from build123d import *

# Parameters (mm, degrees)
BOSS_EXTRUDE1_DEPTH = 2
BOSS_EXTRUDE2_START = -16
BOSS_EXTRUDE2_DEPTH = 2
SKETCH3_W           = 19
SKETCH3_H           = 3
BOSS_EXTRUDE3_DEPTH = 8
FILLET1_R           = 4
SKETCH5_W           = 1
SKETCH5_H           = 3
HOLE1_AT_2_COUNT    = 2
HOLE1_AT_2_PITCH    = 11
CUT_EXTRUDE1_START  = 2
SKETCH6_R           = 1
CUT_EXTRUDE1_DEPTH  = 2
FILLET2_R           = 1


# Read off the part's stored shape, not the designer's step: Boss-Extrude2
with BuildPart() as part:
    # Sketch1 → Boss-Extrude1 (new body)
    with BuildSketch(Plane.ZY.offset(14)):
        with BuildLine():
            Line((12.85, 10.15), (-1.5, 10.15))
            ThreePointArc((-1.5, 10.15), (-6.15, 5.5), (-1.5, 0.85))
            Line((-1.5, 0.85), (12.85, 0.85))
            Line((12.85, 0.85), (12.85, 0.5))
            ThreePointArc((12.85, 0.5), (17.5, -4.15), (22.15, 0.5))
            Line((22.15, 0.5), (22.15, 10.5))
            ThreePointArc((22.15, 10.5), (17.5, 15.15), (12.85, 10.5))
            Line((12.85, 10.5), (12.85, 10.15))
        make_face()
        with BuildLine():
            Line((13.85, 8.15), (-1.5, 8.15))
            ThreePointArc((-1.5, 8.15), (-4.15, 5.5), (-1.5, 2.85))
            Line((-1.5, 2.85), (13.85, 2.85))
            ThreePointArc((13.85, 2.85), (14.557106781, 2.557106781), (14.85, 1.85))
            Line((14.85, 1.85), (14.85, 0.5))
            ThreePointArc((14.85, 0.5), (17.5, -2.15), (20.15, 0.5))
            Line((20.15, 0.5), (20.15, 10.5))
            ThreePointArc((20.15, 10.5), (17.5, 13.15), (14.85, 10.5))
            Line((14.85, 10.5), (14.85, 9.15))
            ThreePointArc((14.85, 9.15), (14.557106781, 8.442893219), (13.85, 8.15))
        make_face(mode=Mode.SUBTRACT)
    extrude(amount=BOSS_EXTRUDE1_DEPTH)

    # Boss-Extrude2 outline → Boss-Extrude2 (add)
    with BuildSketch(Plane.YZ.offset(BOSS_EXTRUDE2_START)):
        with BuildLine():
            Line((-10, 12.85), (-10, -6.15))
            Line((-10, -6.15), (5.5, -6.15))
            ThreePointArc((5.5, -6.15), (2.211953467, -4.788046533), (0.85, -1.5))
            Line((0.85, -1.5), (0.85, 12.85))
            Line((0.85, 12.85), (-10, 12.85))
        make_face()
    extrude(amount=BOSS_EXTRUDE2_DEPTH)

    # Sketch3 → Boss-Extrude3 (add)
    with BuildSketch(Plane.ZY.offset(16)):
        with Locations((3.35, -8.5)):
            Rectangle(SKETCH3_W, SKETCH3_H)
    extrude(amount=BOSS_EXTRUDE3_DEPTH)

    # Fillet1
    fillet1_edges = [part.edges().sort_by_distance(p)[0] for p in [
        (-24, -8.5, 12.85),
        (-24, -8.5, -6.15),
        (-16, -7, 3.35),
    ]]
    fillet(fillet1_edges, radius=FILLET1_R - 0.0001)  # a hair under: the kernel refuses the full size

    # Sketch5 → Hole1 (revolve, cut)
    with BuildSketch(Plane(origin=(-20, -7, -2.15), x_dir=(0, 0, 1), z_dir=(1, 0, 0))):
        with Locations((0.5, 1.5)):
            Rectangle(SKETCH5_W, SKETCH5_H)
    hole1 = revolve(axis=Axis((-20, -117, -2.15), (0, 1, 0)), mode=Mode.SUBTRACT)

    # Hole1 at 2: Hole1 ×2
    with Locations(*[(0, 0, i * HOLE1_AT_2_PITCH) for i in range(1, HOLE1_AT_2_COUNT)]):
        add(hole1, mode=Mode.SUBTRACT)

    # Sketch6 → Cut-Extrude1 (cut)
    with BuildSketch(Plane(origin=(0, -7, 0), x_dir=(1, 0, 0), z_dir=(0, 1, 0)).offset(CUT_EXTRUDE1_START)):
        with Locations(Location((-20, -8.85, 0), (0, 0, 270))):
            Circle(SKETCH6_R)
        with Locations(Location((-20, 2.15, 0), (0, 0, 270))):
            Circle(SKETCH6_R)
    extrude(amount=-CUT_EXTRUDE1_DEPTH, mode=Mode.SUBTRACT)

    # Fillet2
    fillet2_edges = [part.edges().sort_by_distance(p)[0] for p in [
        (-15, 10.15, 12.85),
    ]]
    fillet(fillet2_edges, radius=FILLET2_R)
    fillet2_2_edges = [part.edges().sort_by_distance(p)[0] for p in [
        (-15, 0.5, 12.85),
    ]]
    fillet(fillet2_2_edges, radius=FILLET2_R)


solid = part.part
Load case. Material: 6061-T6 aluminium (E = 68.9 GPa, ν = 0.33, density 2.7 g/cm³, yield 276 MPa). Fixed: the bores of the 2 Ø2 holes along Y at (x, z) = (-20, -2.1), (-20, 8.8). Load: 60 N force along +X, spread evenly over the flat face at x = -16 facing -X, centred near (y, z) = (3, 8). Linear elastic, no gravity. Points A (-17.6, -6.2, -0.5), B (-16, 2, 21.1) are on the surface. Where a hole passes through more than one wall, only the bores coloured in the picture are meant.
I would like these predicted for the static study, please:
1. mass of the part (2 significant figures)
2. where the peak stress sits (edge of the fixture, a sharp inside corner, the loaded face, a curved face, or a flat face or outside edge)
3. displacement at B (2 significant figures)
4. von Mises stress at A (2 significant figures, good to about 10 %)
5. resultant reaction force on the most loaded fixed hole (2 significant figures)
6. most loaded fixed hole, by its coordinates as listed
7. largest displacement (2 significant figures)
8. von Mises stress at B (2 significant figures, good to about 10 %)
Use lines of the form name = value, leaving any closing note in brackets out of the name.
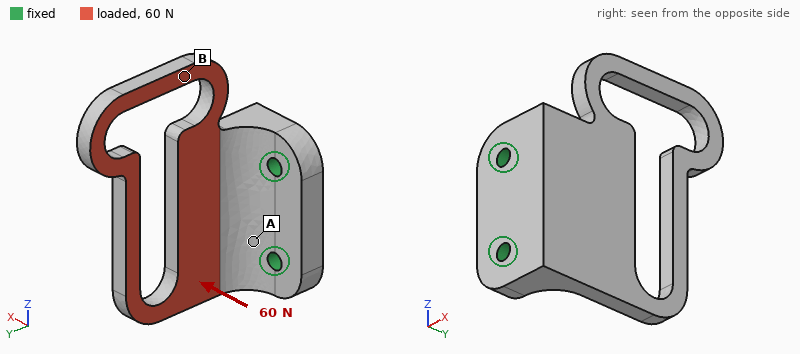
mass of the part = 3.3 g
where the peak stress sits = a curved face
displacement at B = 0.14 mm
von Mises stress at A = 17 MPa
resultant reaction force on the most loaded fixed hole = 52 N
most loaded fixed hole, by its coordinates as listed = (-20, 8.8)
largest displacement = 0.38 mm
von Mises stress at B = 42 MPa
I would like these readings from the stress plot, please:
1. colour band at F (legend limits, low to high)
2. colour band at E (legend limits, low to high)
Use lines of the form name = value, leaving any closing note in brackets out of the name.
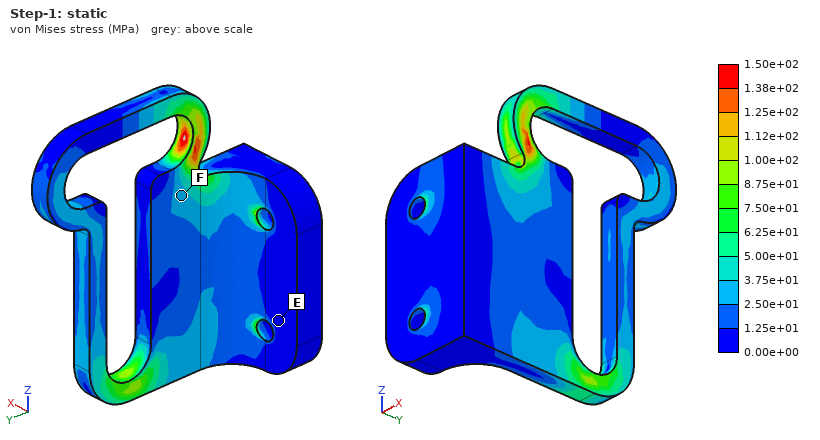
colour band at F = 2.50e+01 to 3.75e+01 MPa
colour band at E = 0.00e+00 to 1.25e+01 MPa
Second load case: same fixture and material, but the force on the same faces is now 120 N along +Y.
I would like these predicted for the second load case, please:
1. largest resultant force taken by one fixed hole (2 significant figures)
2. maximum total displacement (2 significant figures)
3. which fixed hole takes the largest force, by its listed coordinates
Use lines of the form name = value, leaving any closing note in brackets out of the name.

largest resultant force taken by one fixed hole = 100 N
maximum total displacement = 86 µm
which fixed hole takes the largest force, by its listed coordinates = (-20, 8.8)
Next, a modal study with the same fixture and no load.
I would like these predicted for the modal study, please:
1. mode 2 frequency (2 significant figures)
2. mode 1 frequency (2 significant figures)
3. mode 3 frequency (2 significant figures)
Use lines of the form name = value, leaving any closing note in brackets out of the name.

mode 2 frequency = 6600 Hz
mode 1 frequency = 2200 Hz
mode 3 frequency = 6800 Hz
